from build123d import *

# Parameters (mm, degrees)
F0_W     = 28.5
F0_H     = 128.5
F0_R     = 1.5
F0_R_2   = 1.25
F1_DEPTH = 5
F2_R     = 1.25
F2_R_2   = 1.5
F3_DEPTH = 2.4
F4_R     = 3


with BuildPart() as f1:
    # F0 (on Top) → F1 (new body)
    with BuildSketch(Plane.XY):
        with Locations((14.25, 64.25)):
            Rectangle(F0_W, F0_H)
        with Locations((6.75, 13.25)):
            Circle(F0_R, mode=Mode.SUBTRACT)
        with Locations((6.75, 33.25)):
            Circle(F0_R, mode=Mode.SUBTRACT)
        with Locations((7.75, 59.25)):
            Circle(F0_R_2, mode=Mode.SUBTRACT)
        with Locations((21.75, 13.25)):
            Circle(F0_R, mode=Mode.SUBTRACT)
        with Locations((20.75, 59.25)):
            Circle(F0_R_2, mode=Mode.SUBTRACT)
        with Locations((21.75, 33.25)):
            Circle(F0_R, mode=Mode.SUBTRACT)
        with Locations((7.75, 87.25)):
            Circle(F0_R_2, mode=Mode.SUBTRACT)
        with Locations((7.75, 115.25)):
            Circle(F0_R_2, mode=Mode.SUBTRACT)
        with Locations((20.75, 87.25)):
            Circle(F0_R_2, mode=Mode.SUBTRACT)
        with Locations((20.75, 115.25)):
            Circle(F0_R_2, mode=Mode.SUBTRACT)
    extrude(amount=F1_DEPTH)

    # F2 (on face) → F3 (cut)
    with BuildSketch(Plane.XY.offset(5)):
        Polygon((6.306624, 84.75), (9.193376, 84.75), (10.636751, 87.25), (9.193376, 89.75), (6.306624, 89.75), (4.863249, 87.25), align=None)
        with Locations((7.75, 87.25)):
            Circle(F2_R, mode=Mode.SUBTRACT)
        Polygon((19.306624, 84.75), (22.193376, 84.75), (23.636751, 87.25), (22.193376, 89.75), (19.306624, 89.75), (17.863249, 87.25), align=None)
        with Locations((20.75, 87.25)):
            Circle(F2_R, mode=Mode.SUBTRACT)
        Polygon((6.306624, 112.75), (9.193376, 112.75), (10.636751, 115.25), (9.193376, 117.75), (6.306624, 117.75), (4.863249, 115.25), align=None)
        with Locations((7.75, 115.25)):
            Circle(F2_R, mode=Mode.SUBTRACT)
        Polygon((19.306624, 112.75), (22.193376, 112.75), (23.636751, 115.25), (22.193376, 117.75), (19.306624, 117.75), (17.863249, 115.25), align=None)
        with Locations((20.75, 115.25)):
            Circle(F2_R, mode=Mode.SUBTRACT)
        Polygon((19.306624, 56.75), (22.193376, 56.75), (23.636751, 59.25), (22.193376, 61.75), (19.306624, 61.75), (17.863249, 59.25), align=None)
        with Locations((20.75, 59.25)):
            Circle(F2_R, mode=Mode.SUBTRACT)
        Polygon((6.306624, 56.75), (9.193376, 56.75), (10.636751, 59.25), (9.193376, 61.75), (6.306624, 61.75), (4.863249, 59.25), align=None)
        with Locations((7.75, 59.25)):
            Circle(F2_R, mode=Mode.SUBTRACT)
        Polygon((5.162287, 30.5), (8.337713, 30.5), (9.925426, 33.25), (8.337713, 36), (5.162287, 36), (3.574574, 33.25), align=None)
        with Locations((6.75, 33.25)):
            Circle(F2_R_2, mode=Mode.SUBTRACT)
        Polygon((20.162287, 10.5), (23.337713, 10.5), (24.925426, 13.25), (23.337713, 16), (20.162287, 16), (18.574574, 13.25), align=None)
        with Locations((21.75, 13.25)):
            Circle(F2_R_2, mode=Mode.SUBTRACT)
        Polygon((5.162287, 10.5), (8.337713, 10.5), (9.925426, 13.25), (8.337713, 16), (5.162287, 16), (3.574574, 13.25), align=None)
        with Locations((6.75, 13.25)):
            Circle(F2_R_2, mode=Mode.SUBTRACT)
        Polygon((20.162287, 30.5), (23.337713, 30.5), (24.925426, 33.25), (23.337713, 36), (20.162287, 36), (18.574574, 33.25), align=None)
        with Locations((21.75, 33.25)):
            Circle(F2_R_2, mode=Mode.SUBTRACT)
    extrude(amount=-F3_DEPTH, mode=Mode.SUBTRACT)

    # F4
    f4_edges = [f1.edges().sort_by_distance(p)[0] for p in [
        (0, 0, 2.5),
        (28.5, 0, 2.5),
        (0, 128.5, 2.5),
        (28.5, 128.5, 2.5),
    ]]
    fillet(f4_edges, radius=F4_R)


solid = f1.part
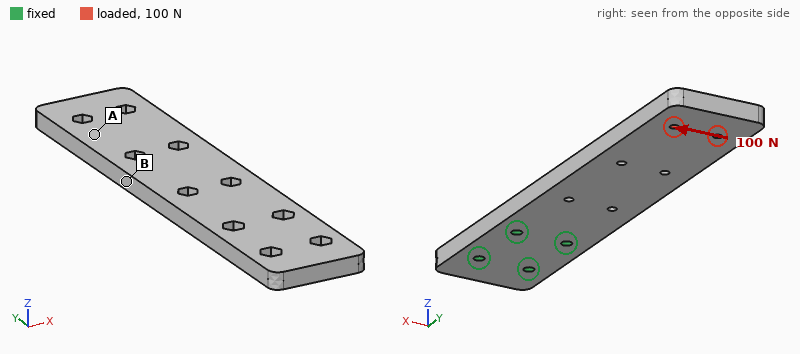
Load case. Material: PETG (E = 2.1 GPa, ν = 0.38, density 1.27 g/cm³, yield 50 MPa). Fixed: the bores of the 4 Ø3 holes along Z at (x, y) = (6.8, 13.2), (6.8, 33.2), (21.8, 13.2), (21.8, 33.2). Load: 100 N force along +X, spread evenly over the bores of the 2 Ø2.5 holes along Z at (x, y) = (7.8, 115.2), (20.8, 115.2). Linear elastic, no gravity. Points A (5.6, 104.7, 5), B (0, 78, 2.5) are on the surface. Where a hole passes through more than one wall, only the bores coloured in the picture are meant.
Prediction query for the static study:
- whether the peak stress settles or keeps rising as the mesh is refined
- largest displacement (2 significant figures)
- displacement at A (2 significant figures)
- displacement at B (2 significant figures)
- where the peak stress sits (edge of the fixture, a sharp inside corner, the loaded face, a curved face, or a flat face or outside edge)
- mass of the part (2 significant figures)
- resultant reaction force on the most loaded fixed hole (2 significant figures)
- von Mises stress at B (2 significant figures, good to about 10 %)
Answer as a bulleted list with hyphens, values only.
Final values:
- keeps rising
- 1.6 mm
- 1.0 mm
- 0.58 mm
- edge of the fixture
- 22 g
- 340 N
- 5.9 MPa
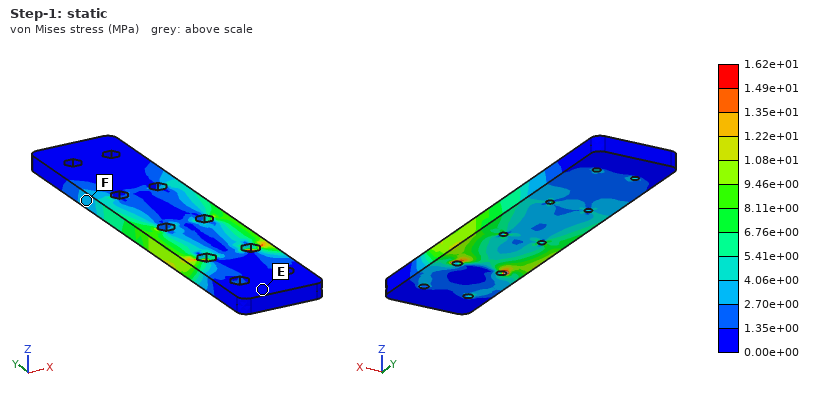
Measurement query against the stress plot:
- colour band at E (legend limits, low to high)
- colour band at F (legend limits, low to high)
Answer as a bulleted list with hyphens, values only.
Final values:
- 0.00e+00 to 1.35e+00 MPa
- 2.70e+00 to 4.06e+00 MPa
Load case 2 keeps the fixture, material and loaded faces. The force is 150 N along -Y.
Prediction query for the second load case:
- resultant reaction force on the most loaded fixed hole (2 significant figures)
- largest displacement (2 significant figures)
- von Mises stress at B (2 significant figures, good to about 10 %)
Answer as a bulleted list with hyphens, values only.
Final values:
- 65 N
- 1.3 mm
- 1.1 MPa
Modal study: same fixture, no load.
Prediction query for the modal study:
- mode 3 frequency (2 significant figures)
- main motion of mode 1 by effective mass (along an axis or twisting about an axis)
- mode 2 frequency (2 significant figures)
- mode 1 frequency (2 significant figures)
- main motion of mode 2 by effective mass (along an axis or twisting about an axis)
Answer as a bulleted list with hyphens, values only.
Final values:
- 660 Hz
- along Z
- 550 Hz
- 110 Hz
- along X
